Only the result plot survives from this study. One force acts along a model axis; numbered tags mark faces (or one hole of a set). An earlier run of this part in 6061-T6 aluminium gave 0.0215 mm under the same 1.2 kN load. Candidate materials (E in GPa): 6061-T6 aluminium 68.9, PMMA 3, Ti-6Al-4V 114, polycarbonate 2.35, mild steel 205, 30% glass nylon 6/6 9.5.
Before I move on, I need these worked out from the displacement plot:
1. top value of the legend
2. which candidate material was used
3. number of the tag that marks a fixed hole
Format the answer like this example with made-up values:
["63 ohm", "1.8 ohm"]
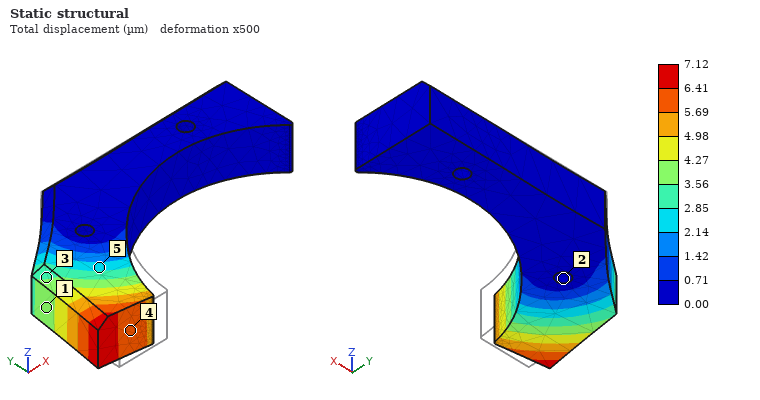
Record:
["7.12 µm", "mild steel", "2"]
